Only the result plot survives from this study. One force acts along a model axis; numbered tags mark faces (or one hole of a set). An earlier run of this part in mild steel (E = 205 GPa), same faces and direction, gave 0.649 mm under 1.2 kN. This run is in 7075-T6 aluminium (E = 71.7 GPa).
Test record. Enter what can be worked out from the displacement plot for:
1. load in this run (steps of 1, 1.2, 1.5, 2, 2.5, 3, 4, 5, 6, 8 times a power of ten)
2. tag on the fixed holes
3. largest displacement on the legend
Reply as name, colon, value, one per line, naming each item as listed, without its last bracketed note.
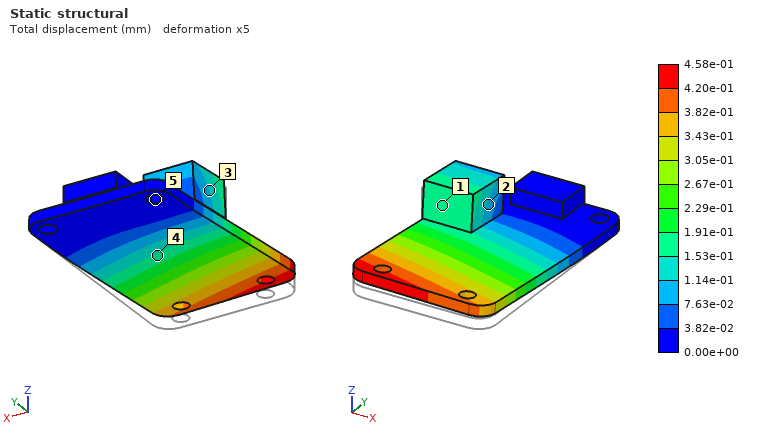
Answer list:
load in this run: 300 N
tag on the fixed holes: 5
largest displacement on the legend: 4.58e-01 mm
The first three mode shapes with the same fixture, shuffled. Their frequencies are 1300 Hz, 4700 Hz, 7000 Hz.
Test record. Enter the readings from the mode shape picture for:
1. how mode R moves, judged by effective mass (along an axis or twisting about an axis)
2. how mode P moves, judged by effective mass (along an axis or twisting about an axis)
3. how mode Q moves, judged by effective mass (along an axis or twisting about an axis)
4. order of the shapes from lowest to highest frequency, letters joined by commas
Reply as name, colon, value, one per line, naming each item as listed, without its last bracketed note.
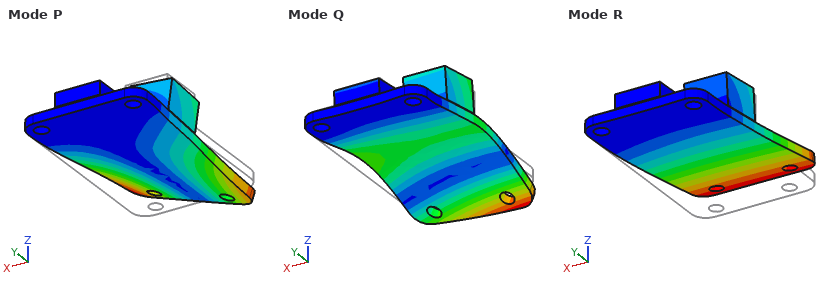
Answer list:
how mode R moves, judged by effective mass: along Z
how mode P moves, judged by effective mass: twisting about Y
how mode Q moves, judged by effective mass: along Z
order of the shapes from lowest to highest frequency, letters joined by commas: R, P, Q
